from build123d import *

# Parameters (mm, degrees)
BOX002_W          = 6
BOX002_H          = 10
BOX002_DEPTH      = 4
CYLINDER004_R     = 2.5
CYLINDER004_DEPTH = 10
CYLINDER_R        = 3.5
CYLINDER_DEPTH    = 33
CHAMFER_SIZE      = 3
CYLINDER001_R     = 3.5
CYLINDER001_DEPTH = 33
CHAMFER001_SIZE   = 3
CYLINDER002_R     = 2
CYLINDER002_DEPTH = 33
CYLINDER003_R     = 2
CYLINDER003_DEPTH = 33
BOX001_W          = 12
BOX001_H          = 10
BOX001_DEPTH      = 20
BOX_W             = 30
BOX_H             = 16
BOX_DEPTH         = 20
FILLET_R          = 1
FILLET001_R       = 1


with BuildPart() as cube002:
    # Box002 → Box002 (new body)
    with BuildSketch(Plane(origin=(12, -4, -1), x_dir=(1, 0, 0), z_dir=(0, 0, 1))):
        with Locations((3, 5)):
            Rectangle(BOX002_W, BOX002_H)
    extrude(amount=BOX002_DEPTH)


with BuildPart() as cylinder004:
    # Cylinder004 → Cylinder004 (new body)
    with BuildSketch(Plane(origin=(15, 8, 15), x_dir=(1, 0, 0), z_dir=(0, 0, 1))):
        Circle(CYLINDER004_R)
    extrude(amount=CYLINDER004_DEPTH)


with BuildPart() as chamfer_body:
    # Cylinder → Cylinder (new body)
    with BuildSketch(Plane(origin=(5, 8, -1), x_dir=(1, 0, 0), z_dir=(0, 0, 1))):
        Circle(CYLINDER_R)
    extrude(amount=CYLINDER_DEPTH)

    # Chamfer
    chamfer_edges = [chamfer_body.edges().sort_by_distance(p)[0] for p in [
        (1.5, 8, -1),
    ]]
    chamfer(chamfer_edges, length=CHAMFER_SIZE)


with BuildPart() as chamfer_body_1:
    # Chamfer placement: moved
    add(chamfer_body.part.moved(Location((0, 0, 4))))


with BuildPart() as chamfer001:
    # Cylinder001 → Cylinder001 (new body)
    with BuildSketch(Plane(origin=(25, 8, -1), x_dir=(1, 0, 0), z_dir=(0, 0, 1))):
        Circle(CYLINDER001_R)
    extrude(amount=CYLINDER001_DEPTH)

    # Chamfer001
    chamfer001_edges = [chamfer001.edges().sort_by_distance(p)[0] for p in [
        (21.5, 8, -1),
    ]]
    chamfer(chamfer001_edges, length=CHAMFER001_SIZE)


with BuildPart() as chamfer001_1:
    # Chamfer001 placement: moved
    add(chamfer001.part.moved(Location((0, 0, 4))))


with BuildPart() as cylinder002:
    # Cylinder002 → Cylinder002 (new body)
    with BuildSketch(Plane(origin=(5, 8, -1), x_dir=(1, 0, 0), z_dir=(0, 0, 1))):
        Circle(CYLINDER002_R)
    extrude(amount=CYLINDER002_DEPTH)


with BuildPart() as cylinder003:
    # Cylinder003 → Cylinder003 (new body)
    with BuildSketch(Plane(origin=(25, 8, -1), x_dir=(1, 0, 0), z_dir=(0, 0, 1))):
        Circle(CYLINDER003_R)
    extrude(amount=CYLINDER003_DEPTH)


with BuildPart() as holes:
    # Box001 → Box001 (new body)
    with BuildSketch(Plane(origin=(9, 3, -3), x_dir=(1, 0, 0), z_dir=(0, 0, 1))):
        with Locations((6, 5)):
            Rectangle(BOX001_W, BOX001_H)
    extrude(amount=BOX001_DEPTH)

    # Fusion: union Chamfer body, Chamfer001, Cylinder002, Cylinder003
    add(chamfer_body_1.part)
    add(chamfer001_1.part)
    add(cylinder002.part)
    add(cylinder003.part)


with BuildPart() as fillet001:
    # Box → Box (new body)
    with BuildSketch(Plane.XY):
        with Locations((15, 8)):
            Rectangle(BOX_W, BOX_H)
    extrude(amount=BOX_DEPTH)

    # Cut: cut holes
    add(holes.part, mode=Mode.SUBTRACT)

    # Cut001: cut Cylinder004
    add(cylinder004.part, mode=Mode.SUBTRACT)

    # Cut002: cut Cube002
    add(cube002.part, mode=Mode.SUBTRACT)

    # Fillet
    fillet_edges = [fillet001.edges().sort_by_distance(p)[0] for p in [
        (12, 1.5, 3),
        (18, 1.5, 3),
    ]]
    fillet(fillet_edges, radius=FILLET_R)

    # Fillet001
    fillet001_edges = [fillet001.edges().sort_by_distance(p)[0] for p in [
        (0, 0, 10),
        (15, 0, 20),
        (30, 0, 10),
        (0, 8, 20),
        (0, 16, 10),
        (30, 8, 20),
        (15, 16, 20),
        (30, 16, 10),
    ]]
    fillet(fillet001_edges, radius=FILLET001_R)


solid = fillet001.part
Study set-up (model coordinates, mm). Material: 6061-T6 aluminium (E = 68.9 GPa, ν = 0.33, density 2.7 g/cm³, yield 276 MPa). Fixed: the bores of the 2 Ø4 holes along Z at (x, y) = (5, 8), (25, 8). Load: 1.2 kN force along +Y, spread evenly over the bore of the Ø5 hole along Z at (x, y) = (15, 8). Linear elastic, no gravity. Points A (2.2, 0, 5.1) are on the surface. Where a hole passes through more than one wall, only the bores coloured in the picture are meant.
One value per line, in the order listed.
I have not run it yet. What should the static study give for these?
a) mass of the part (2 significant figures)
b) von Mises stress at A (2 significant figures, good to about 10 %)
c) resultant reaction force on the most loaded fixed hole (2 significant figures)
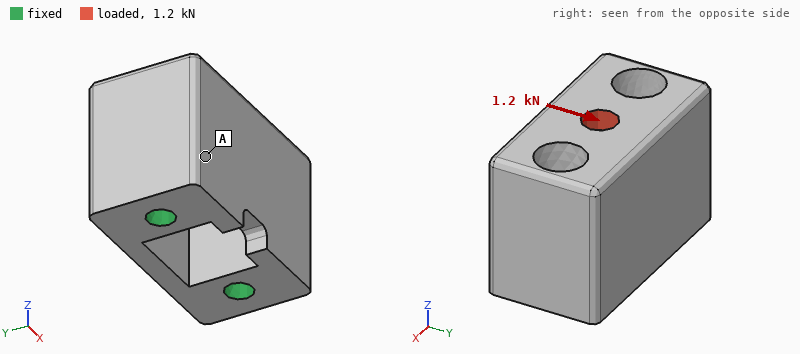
17 g
19 MPa
600 N
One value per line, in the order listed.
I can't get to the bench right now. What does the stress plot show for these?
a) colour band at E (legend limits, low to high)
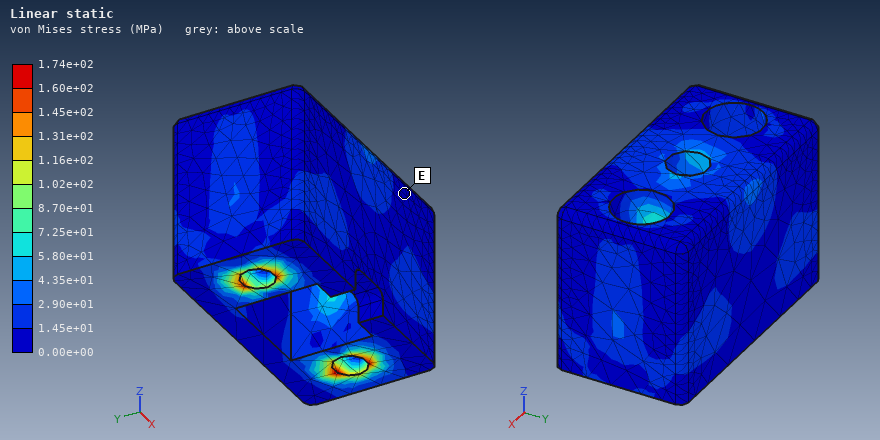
0.00e+00 to 1.45e+01 MPa
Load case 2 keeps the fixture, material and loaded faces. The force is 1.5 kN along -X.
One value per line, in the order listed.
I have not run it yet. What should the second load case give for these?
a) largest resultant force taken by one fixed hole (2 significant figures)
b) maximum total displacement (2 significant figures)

1.2 kN
15 µm
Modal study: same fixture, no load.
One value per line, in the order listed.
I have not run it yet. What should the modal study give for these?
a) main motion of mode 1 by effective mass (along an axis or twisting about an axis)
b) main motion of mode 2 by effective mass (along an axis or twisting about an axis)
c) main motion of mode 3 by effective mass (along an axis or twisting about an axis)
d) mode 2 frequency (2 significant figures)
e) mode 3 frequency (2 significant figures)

along Y
along X
twisting about Z
21 kHz
23 kHz
